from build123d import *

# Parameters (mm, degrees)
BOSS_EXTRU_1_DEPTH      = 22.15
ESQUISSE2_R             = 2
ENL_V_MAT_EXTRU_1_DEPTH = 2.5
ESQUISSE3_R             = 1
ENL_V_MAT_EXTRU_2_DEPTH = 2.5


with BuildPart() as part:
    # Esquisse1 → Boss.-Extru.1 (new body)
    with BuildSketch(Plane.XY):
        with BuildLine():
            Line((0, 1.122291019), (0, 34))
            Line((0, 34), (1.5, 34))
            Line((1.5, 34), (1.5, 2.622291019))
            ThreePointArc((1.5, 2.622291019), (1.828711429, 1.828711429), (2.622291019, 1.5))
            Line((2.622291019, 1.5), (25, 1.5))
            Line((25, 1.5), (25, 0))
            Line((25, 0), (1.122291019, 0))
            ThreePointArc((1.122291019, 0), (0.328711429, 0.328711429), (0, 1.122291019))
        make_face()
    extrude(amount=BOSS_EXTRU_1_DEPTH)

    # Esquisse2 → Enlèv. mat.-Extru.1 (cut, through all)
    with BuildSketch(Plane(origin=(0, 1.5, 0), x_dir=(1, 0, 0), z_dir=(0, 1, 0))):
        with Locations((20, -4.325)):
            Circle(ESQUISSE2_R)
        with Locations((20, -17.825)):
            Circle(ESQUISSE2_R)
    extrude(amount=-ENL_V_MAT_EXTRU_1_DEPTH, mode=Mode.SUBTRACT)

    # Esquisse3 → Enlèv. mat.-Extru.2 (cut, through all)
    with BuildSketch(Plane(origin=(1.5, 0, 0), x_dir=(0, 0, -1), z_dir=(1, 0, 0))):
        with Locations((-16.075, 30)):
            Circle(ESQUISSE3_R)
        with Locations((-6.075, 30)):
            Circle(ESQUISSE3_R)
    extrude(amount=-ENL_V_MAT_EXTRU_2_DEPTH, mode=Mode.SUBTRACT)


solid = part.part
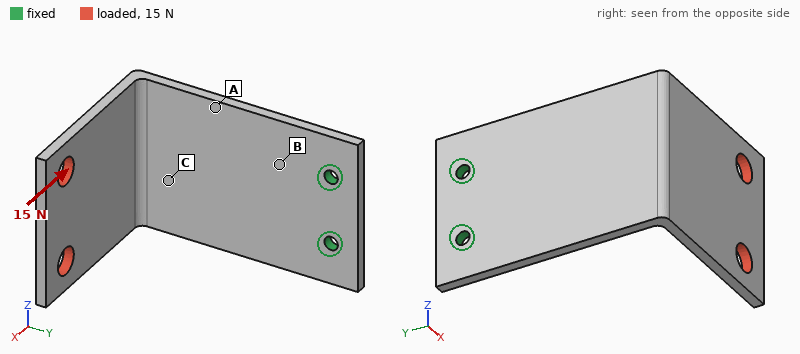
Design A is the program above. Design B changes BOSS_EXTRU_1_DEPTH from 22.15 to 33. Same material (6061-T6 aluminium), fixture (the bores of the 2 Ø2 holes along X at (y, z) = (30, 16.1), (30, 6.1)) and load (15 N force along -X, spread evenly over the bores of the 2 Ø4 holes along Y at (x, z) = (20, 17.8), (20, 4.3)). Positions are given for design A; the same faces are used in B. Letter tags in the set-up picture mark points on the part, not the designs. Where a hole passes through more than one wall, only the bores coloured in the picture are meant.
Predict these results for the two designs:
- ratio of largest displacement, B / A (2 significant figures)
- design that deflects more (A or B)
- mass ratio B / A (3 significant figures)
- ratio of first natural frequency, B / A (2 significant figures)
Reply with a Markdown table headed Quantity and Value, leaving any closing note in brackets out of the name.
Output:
| Quantity | Value |
|---|---|
| ratio of largest displacement, B / A | 0.79 |
| design that deflects more | A |
| mass ratio B / A | 1.50 |
| ratio of first natural frequency, B / A | 0.92 |
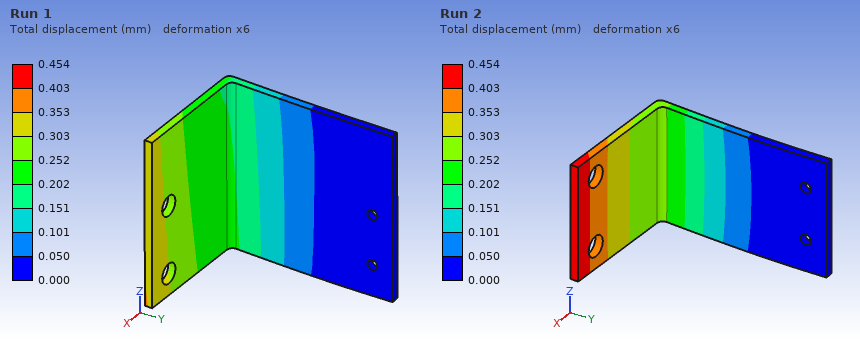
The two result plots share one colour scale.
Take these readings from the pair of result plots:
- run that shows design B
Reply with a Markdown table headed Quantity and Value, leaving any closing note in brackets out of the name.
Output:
| Quantity | Value |
|---|---|
| run that shows design B | Run 1 |
